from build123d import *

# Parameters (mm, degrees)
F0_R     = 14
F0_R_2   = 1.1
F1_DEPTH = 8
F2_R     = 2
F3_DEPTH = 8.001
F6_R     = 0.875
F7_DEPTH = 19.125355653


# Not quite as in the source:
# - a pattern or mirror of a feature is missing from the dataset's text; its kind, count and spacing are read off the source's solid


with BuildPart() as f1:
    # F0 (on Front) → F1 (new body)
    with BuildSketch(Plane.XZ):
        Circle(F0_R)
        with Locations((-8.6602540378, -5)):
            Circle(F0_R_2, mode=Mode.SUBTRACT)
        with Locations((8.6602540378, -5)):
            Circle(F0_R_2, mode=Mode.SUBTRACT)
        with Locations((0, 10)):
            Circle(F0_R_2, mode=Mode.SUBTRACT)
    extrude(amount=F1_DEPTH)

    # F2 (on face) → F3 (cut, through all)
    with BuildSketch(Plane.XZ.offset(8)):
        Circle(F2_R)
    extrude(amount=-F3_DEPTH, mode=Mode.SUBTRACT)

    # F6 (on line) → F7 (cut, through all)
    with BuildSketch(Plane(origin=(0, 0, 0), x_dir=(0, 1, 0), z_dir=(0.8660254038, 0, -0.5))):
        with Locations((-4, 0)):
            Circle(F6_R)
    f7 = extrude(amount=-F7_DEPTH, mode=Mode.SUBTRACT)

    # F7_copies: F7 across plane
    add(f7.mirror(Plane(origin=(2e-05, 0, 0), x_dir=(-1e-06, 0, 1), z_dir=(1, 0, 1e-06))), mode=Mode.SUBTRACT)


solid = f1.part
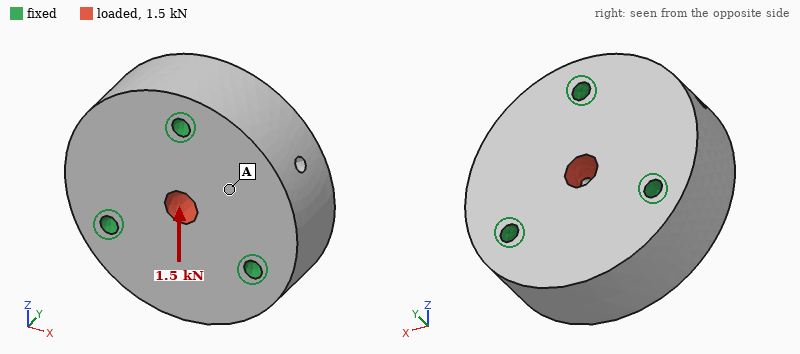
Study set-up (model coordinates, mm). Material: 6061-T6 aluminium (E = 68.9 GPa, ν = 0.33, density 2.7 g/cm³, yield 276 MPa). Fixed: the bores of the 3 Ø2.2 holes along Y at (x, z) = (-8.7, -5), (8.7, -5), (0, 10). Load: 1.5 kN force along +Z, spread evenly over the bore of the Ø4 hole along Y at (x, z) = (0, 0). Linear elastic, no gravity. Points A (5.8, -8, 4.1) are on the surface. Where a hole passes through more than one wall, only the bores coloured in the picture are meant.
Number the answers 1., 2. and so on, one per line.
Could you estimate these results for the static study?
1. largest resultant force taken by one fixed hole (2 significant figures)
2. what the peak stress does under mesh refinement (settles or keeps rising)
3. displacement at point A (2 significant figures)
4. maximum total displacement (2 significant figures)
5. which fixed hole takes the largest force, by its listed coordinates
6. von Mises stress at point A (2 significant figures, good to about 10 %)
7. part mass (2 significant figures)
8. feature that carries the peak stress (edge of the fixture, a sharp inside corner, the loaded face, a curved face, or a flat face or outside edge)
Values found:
1. 540 N
2. keeps rising
3. 0.73 µm
4. 2.0 µm
5. (0, 10)
6. 3.7 MPa
7. 13 g
8. a sharp inside corner
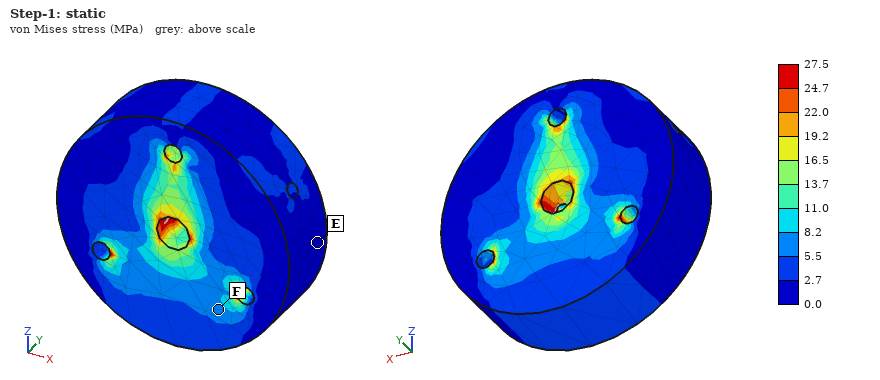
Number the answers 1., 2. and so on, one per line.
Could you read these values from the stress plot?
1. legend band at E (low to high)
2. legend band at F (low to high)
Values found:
1. 0.0 to 2.7 MPa
2. 5.5 to 8.2 MPa
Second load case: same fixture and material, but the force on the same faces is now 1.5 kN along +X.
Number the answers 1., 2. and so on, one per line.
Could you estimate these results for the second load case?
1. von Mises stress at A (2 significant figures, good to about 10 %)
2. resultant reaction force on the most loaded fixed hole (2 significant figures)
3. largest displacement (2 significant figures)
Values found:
1. 5.4 MPa
2. 530 N
3. 2.0 µm
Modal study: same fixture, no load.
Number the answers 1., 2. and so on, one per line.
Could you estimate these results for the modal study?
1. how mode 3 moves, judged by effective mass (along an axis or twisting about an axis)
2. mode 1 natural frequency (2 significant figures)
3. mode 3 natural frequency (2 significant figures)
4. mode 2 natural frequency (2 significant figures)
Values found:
1. along Y
2. 47 kHz
3. 52 kHz
4. 47 kHz
